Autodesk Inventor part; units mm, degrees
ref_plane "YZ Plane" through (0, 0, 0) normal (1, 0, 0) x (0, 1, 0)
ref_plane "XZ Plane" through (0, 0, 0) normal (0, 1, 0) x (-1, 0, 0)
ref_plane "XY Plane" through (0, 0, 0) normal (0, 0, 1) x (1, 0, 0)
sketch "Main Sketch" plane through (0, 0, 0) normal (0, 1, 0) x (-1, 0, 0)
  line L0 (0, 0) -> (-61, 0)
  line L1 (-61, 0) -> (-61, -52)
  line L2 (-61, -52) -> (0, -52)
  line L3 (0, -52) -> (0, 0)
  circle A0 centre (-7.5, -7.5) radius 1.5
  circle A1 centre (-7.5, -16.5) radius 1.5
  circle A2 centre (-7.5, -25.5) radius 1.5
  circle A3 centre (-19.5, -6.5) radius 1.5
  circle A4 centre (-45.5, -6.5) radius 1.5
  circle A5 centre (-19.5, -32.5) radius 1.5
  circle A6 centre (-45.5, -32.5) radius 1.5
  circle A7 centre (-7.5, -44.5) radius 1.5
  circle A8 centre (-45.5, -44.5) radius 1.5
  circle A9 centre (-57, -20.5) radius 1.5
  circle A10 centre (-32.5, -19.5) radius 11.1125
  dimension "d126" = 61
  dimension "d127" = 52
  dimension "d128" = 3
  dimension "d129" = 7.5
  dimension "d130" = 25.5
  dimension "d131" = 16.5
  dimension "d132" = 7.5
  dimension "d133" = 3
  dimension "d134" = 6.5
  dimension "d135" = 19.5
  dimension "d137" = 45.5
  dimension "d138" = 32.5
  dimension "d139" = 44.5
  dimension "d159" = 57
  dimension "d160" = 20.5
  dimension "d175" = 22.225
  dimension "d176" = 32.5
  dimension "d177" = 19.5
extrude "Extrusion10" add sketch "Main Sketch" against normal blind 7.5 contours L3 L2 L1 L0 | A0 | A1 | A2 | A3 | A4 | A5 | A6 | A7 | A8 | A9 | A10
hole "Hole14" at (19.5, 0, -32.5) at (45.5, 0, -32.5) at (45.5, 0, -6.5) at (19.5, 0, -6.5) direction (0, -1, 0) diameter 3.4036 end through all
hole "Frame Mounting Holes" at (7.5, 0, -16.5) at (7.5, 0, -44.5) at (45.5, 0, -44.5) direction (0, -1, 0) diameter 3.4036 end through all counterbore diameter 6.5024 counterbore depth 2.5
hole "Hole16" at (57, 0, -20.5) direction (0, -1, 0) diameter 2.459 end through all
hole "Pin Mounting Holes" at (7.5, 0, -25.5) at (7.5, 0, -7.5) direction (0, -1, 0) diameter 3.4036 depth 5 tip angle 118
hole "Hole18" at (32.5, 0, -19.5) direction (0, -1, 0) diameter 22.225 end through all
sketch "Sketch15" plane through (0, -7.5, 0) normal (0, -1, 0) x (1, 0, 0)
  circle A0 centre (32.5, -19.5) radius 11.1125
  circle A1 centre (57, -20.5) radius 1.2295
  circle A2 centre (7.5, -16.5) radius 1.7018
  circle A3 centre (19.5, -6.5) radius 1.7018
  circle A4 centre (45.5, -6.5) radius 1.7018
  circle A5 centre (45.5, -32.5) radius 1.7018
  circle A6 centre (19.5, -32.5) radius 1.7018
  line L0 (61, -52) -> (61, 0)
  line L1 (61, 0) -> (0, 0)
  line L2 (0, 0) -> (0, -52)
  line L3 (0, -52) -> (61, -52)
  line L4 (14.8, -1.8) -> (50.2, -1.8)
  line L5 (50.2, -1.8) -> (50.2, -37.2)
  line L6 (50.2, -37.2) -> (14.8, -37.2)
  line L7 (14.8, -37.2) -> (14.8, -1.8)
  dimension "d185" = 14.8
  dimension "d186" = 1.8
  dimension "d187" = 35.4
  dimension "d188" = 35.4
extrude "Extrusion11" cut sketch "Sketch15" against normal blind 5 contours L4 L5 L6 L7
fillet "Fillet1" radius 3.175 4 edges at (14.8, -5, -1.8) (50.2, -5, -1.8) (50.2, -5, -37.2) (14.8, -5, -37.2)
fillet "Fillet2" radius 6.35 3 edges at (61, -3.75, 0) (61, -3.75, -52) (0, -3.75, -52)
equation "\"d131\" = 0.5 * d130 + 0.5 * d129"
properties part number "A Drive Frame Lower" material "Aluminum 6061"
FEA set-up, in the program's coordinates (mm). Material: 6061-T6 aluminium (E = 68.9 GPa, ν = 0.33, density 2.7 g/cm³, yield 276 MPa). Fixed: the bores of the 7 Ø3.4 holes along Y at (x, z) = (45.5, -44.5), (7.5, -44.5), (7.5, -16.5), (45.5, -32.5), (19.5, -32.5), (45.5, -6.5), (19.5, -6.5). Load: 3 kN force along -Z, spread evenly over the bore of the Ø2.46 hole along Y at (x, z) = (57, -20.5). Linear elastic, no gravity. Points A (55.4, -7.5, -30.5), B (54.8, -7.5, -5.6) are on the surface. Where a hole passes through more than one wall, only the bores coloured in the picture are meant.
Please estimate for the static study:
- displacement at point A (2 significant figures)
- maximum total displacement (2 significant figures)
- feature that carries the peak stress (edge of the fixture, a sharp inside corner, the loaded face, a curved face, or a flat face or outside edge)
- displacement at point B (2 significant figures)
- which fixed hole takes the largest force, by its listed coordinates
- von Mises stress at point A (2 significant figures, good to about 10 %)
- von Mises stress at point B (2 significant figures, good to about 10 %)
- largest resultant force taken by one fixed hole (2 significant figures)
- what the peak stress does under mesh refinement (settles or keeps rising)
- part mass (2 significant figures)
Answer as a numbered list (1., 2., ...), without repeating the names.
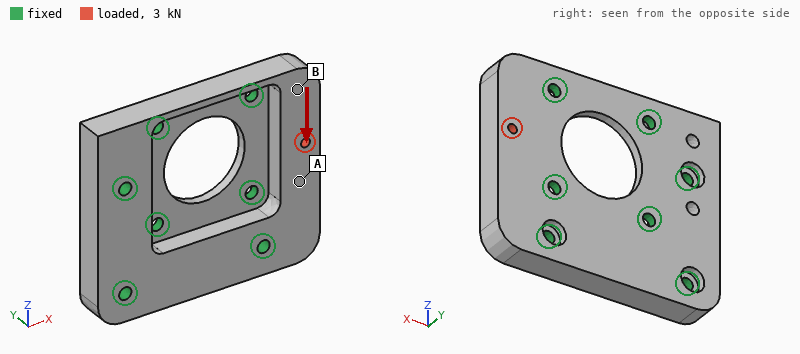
1. 9.2 µm
2. 14 µm
3. edge of the fixture
4. 10 µm
5. (45.5, -6.5)
6. 24 MPa
7. 8.8 MPa
8. 1.3 kN
9. keeps rising
10. 43 g
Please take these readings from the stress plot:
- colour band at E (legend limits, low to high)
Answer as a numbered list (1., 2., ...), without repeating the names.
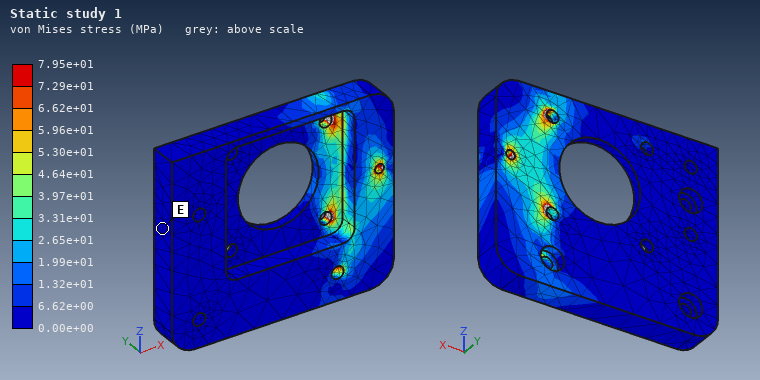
1. 0.00e+00 to 6.62e+00 MPa
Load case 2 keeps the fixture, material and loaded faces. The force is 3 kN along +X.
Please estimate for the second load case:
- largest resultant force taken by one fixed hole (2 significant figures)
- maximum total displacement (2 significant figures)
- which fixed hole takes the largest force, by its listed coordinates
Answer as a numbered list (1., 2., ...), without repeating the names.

1. 1.6 kN
2. 51 µm
3. (45.5, -6.5)
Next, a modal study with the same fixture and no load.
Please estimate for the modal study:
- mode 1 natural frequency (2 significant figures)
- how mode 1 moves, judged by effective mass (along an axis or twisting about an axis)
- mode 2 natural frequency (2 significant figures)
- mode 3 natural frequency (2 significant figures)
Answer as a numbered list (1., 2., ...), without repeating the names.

1. 9600 Hz
2. along Y
3. 17 kHz
4. 19 kHz
